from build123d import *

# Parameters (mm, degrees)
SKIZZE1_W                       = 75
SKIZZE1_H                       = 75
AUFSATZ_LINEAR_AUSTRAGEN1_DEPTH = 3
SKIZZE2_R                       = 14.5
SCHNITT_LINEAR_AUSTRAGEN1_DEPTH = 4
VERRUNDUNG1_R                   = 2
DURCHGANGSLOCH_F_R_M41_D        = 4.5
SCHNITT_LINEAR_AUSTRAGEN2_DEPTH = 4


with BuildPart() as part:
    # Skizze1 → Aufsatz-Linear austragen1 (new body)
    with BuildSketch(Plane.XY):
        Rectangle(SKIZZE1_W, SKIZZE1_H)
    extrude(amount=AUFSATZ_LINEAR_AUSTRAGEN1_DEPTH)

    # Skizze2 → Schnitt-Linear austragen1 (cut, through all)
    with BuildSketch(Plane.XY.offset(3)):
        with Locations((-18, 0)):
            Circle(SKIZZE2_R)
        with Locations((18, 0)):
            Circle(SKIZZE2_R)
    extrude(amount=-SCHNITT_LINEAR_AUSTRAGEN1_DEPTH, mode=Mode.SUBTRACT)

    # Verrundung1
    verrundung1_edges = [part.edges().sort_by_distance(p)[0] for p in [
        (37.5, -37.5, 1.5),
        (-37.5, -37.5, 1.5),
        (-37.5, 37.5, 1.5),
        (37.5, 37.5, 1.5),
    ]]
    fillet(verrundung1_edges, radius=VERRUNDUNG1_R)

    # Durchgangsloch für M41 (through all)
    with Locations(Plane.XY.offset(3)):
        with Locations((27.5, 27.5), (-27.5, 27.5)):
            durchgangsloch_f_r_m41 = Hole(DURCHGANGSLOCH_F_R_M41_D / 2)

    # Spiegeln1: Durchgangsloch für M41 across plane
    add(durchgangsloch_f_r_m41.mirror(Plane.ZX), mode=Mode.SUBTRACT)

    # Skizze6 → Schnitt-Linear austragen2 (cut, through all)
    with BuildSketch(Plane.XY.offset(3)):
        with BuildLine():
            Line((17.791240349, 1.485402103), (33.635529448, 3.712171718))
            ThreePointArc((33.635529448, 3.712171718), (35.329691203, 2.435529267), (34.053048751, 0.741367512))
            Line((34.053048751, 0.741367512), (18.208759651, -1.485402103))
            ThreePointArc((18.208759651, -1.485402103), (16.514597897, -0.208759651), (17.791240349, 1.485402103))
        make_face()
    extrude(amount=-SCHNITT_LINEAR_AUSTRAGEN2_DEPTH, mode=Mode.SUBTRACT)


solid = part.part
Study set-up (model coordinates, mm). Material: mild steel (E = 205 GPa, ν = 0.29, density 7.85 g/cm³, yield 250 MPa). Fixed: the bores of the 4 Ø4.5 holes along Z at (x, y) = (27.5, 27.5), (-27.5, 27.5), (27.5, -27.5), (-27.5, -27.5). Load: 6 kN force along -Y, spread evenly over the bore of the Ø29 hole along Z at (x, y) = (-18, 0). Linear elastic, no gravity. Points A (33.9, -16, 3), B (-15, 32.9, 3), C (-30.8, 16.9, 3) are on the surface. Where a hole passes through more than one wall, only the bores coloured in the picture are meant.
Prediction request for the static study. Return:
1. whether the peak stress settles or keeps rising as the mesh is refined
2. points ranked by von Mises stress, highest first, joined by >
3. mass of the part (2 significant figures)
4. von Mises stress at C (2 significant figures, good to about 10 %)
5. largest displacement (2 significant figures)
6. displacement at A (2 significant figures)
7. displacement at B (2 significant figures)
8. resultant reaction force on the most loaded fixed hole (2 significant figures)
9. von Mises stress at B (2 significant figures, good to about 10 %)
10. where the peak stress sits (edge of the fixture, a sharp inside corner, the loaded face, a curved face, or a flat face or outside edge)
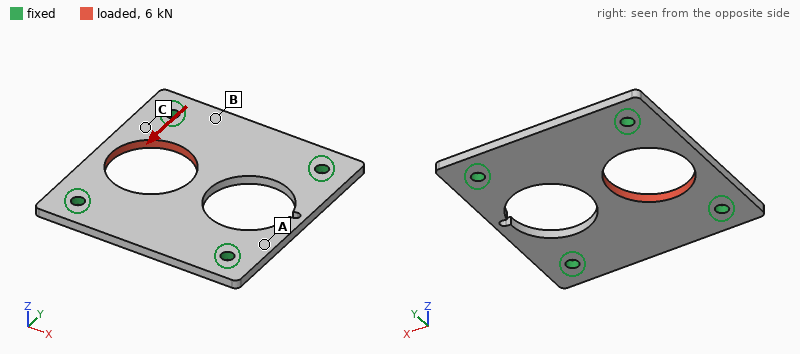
keeps rising
C > B > A
100 g
35 MPa
6.8 µm
1.2 µm
4.0 µm
2.4 kN
18 MPa
edge of the fixture
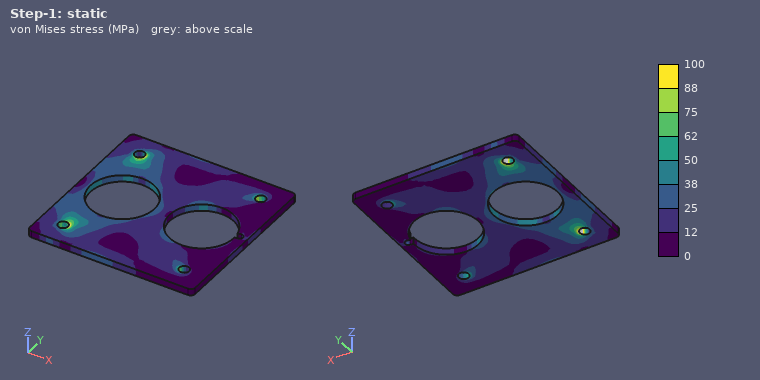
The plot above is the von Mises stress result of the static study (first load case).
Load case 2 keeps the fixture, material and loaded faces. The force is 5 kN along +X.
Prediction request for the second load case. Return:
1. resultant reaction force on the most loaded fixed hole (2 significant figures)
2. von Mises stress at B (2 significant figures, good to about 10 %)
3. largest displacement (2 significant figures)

1.6 kN
14 MPa
16 µm
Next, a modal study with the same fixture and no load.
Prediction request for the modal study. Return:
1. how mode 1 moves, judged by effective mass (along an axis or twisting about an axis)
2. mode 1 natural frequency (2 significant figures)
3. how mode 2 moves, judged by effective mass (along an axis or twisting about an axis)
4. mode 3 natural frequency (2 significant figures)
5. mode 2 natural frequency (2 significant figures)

along Z
4100 Hz
twisting about X
6100 Hz
5400 Hz
